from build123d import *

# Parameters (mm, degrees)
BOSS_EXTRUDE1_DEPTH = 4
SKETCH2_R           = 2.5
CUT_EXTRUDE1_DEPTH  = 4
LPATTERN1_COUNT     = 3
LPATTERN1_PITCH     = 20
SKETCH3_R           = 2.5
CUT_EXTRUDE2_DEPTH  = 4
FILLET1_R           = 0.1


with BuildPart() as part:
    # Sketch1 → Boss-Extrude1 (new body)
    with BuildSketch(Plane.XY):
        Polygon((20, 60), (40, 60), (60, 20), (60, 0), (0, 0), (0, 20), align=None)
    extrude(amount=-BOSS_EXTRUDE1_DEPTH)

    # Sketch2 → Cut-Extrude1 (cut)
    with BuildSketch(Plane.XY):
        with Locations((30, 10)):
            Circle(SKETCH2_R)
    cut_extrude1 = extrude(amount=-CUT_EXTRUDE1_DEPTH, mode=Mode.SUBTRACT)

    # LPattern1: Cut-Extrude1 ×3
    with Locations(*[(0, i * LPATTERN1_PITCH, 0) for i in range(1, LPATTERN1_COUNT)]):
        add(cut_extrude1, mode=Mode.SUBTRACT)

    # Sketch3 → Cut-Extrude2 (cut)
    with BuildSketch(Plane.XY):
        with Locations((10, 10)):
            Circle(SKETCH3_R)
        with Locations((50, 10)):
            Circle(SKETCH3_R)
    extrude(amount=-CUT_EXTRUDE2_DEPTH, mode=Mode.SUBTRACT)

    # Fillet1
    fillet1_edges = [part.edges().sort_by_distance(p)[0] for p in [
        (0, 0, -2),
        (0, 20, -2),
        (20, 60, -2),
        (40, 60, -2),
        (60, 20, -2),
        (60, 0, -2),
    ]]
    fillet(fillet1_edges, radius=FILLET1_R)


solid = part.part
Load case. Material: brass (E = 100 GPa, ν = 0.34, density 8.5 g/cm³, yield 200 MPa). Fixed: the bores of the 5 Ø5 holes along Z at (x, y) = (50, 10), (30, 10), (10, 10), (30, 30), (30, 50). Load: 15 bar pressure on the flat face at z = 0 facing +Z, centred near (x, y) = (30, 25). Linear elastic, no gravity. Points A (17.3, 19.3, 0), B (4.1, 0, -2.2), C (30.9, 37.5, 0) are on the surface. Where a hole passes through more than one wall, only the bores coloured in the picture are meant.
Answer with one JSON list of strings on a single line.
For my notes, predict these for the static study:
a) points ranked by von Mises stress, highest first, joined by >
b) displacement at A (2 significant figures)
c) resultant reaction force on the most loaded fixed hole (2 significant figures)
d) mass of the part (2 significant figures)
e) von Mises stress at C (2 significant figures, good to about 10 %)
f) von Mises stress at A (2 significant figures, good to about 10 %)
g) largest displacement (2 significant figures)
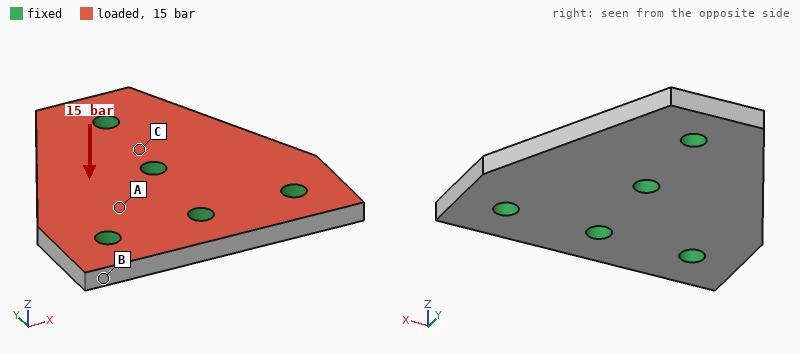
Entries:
["C > A > B", "5.7 µm", "1.0 kN", "92 g", "42 MPa", "24 MPa", "32 µm"]
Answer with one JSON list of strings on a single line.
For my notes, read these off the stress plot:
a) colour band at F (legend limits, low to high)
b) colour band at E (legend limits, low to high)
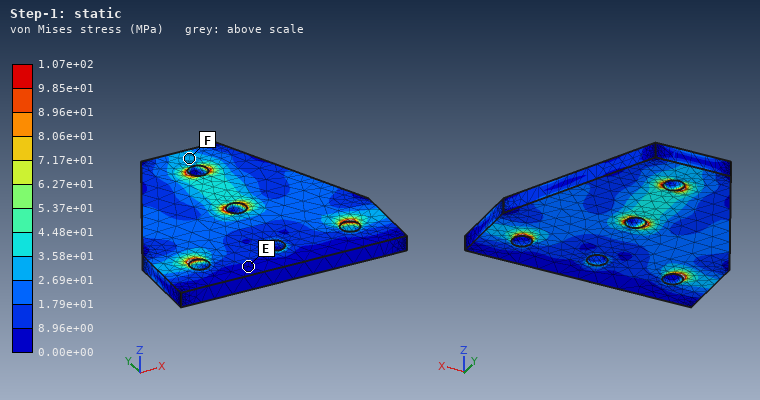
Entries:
["2.69e+01 to 3.58e+01 MPa", "0.00e+00 to 8.96e+00 MPa"]
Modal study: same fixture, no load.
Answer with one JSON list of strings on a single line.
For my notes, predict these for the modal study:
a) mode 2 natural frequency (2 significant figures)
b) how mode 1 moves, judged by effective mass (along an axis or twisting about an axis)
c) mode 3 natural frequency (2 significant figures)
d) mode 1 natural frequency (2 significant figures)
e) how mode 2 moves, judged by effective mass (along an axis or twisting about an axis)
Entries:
["8000 Hz", "twisting about Y", "14 kHz", "7500 Hz", "along Z"]
